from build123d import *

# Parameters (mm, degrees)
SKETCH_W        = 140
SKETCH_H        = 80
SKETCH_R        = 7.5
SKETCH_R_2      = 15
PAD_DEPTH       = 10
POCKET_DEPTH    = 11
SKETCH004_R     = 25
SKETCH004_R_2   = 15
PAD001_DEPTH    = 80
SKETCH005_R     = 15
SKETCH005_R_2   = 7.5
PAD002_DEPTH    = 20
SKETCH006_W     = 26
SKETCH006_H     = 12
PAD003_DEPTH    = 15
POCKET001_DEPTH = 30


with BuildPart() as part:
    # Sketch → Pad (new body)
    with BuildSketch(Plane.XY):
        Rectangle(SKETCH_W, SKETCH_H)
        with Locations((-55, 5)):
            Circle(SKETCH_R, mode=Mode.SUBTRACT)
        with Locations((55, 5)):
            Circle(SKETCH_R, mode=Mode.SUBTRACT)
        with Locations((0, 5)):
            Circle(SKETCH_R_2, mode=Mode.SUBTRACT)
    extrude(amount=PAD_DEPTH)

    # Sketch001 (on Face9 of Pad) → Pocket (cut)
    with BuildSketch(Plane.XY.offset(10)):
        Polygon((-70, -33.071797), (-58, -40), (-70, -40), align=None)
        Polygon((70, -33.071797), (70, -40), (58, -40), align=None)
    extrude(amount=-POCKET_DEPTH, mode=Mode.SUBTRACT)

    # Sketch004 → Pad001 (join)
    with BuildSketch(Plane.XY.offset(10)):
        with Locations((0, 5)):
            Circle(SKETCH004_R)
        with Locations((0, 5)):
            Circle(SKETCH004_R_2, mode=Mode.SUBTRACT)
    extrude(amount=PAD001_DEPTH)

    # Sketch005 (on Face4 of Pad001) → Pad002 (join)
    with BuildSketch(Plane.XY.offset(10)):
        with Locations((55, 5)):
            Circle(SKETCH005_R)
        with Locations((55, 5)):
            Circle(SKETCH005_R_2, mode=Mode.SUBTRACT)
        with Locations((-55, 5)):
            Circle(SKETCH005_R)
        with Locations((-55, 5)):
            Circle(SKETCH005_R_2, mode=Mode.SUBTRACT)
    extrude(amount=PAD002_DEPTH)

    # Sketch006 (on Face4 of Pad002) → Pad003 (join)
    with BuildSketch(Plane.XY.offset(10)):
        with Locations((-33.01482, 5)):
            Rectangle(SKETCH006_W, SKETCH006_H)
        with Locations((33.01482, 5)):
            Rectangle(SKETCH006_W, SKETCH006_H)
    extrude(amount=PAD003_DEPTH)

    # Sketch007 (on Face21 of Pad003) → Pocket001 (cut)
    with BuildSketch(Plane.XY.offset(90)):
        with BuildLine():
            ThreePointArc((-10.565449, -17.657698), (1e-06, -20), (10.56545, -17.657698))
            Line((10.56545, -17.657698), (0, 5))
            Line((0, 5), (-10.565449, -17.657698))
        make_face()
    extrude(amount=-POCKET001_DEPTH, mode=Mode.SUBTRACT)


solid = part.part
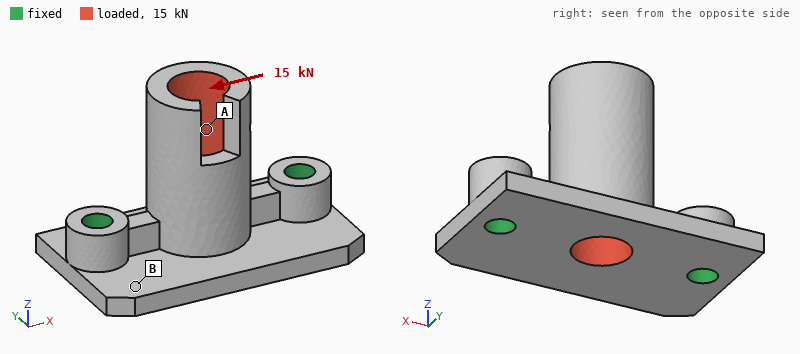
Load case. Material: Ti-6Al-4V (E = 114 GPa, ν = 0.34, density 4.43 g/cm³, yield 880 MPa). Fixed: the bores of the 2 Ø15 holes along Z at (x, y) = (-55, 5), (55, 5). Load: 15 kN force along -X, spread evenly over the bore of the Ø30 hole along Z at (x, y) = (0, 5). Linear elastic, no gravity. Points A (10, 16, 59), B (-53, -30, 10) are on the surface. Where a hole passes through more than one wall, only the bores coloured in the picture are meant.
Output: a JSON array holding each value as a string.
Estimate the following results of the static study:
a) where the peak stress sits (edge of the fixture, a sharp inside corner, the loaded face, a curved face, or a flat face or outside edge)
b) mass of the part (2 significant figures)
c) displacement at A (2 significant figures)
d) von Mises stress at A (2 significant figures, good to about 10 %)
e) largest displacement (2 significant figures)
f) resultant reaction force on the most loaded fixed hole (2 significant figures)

["a flat face or outside edge", "990 g", "45 µm", "17 MPa", "81 µm", "9.8 kN"]
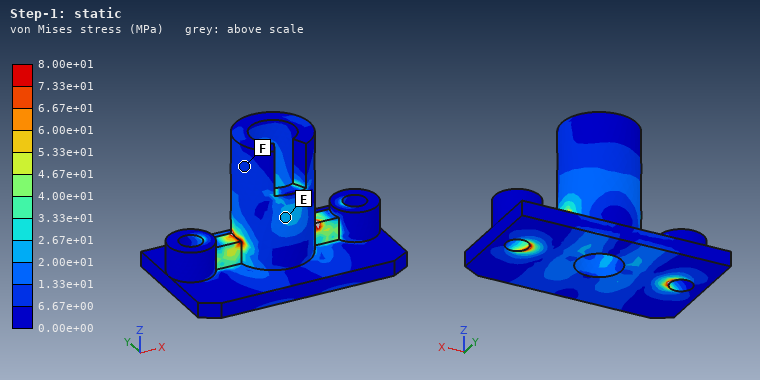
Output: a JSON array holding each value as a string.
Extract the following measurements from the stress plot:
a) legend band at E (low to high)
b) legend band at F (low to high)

["2.00e+01 to 2.67e+01 MPa", "6.67e+00 to 1.33e+01 MPa"]
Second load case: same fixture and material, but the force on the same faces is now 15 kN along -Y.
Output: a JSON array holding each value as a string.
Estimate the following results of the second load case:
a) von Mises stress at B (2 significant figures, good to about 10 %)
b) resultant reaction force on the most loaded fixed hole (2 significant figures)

["34 MPa", "7.5 kN"]
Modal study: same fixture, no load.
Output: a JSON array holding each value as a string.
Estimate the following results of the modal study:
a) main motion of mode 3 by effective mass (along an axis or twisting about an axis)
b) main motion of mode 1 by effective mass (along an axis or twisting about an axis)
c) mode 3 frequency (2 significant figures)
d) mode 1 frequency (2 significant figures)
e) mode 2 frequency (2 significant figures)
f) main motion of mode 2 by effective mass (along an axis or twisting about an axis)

["along Z", "along Y", "4900 Hz", "1700 Hz", "3800 Hz", "along X"]
